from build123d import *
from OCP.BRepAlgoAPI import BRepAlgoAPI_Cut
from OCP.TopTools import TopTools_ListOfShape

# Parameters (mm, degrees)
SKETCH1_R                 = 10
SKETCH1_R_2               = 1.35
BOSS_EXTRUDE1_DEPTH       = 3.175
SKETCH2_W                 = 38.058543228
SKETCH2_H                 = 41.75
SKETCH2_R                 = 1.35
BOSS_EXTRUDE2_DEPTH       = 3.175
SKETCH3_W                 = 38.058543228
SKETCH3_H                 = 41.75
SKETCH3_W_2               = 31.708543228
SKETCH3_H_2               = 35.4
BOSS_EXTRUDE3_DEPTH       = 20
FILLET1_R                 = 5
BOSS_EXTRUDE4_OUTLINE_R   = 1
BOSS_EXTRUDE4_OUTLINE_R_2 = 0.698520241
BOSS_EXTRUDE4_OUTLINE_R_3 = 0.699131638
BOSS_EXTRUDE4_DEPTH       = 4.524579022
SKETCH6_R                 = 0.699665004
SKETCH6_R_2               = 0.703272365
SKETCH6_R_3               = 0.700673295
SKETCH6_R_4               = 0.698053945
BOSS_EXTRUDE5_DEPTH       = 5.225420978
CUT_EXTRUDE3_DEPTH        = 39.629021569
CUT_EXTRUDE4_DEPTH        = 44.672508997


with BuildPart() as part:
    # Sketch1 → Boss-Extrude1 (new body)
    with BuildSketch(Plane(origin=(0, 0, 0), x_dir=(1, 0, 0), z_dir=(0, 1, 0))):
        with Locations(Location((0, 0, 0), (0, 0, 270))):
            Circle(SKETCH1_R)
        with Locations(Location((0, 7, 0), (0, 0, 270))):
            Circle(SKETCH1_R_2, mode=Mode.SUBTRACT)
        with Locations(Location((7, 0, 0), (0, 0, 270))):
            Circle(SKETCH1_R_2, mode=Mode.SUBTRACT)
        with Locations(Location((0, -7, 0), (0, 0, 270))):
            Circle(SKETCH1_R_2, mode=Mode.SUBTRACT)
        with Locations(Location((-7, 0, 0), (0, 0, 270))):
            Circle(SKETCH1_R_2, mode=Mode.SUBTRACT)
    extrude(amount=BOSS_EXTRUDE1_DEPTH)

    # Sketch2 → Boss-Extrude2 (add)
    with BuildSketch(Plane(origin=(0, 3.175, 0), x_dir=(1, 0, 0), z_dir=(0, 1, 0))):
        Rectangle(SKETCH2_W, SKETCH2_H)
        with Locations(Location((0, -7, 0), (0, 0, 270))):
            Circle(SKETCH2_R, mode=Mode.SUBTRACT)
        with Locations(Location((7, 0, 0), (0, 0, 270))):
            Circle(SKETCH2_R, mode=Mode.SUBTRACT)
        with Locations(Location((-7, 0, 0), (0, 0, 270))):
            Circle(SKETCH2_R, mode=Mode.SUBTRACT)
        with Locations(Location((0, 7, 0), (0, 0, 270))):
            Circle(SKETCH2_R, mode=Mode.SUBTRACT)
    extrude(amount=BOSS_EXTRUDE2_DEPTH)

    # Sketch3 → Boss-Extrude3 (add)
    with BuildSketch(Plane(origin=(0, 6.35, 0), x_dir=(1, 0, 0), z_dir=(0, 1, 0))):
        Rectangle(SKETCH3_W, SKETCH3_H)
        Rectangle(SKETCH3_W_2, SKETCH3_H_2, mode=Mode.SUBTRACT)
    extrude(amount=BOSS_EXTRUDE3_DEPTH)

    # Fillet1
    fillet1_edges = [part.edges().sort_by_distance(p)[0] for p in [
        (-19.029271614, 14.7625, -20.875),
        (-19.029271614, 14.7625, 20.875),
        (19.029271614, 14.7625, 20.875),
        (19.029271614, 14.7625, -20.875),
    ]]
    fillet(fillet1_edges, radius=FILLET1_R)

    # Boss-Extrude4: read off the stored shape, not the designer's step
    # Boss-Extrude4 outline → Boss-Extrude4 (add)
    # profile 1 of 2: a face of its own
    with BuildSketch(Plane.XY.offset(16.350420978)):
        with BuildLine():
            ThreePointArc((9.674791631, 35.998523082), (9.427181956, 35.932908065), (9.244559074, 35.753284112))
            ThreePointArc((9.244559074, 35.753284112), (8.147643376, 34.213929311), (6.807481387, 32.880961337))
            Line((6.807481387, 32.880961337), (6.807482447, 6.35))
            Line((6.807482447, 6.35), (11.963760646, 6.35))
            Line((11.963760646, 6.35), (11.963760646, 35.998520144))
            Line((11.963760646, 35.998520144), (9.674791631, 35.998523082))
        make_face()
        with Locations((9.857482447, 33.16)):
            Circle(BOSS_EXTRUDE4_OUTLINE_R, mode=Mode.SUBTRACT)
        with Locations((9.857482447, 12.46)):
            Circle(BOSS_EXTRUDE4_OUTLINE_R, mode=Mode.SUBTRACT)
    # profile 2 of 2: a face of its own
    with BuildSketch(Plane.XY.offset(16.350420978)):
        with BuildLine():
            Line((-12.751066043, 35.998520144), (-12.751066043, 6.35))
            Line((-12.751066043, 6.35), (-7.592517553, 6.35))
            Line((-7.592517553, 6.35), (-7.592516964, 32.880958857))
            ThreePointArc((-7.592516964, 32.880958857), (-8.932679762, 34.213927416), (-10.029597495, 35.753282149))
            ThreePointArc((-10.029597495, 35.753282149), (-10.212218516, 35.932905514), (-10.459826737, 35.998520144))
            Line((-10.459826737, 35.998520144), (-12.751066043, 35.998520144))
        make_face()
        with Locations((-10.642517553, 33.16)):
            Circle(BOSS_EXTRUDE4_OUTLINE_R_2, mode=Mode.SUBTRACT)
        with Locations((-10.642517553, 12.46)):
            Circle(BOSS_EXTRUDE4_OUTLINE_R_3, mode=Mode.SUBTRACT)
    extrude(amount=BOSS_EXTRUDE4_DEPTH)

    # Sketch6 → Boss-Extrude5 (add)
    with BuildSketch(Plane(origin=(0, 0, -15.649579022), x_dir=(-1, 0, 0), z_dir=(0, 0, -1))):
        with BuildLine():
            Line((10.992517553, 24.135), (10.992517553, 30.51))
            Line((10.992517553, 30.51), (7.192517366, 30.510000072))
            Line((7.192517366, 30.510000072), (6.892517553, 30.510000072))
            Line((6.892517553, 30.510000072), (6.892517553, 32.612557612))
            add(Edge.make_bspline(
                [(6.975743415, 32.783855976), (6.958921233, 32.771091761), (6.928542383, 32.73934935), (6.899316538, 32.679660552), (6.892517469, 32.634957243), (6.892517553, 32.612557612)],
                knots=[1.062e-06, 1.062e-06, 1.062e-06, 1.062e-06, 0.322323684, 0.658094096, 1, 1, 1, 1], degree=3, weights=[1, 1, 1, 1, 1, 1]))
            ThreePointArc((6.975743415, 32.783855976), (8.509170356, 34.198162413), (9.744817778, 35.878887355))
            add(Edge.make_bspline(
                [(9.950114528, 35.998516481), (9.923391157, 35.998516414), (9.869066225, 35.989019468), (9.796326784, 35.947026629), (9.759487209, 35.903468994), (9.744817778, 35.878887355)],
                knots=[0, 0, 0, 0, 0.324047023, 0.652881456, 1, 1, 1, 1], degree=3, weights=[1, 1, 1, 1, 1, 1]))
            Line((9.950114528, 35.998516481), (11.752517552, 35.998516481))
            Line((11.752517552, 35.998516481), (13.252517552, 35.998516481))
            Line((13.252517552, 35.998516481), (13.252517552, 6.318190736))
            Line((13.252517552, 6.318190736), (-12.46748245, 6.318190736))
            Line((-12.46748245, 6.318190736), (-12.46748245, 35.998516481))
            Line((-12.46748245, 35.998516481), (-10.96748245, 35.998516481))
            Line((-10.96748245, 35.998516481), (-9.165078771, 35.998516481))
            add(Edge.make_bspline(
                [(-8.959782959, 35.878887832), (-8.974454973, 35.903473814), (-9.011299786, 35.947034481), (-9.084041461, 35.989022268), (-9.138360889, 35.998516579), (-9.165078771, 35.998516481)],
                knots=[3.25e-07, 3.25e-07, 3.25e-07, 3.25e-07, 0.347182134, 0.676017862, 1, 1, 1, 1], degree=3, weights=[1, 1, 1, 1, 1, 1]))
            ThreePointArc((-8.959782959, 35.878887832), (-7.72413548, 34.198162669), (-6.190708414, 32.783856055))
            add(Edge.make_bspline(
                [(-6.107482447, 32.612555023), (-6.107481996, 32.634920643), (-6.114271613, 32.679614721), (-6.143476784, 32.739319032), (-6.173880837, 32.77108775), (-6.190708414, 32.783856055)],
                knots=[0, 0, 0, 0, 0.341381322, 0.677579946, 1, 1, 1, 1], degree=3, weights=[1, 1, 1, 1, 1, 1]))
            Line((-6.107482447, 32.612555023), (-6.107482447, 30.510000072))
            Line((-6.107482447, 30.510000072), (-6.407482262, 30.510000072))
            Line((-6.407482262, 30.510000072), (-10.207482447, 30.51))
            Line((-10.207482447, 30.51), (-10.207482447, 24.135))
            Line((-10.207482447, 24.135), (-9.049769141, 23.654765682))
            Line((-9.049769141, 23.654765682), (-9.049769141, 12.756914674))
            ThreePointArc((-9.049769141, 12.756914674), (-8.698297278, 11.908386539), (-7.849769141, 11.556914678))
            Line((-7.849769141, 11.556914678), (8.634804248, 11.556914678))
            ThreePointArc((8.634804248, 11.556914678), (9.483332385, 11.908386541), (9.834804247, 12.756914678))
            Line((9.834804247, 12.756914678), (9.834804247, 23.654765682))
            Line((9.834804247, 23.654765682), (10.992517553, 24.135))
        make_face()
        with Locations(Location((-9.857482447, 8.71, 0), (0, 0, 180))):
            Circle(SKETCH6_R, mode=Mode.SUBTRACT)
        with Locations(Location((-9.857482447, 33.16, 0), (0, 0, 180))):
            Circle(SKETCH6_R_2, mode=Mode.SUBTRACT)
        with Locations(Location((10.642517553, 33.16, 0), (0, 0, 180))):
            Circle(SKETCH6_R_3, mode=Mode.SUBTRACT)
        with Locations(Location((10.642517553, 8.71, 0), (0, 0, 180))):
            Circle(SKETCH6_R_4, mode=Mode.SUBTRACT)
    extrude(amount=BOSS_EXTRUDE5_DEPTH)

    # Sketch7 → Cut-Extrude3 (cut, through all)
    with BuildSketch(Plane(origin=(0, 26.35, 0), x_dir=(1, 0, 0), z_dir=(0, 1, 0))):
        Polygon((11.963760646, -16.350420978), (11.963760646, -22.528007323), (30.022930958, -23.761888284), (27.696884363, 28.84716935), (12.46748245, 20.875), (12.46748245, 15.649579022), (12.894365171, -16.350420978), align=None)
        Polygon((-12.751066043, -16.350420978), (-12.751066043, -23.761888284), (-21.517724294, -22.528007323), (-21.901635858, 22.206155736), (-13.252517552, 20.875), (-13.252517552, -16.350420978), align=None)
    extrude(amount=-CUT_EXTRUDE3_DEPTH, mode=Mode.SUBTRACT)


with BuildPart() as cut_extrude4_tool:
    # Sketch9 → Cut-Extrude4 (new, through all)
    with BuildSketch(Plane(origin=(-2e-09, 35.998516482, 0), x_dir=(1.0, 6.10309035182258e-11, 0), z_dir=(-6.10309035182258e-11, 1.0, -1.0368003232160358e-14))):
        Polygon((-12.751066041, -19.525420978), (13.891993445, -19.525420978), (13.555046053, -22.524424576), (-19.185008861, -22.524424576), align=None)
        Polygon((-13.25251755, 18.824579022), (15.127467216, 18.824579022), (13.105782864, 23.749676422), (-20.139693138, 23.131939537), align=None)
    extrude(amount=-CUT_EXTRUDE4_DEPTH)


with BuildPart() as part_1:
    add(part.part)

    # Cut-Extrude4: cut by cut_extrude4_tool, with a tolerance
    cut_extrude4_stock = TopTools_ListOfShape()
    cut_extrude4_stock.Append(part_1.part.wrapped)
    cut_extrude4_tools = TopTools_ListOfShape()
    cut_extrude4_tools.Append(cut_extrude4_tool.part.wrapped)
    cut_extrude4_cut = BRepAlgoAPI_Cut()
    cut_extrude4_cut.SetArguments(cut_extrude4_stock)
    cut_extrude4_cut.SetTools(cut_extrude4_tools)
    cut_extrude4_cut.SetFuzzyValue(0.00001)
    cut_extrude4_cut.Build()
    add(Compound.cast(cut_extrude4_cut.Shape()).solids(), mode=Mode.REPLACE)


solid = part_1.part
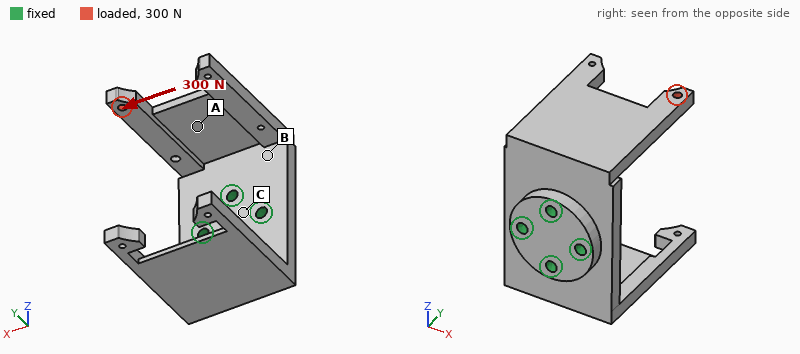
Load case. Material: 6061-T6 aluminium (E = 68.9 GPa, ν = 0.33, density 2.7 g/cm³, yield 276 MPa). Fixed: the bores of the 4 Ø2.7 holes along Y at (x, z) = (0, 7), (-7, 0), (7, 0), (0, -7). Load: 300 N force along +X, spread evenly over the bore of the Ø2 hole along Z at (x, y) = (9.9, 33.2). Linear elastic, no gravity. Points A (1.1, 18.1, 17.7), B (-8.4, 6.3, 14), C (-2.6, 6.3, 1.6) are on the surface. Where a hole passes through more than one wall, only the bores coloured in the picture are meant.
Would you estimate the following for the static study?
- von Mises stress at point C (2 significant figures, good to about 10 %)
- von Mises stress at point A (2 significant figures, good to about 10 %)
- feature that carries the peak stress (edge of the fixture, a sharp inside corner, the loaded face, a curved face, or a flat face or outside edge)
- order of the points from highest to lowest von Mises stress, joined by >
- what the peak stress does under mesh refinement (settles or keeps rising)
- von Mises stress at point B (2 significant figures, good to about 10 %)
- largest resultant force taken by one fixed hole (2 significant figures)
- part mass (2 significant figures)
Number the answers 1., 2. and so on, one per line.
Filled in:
1. 17 MPa
2. 55 MPa
3. edge of the fixture
4. B > A > C
5. keeps rising
6. 91 MPa
7. 310 N
8. 18 g
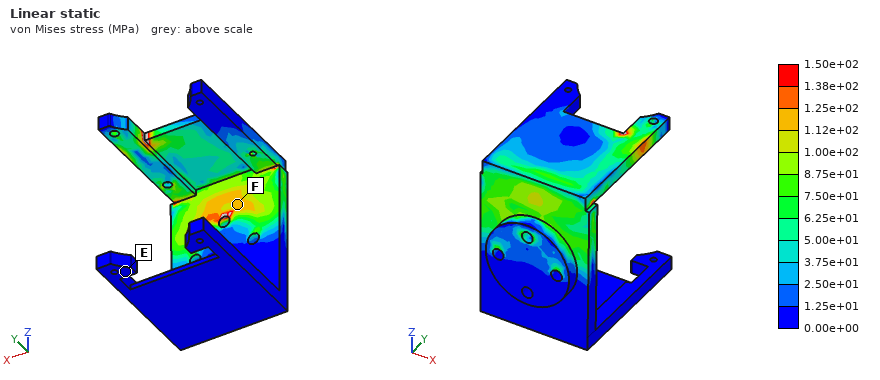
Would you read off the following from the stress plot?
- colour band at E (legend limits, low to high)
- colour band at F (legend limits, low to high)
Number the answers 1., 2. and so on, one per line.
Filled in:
1. 0.00e+00 to 1.25e+01 MPa
2. 1.12e+02 to 1.25e+02 MPa
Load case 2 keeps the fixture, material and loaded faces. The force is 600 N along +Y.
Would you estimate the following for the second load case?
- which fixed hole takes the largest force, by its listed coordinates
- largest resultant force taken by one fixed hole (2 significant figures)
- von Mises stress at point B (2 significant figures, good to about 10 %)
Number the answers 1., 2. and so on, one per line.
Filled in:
1. (0, 7)
2. 800 N
3. 82 MPa
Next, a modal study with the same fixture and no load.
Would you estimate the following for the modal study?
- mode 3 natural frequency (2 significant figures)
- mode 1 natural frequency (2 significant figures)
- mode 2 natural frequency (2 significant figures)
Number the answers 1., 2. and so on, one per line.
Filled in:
1. 3200 Hz
2. 2300 Hz
3. 2500 Hz
